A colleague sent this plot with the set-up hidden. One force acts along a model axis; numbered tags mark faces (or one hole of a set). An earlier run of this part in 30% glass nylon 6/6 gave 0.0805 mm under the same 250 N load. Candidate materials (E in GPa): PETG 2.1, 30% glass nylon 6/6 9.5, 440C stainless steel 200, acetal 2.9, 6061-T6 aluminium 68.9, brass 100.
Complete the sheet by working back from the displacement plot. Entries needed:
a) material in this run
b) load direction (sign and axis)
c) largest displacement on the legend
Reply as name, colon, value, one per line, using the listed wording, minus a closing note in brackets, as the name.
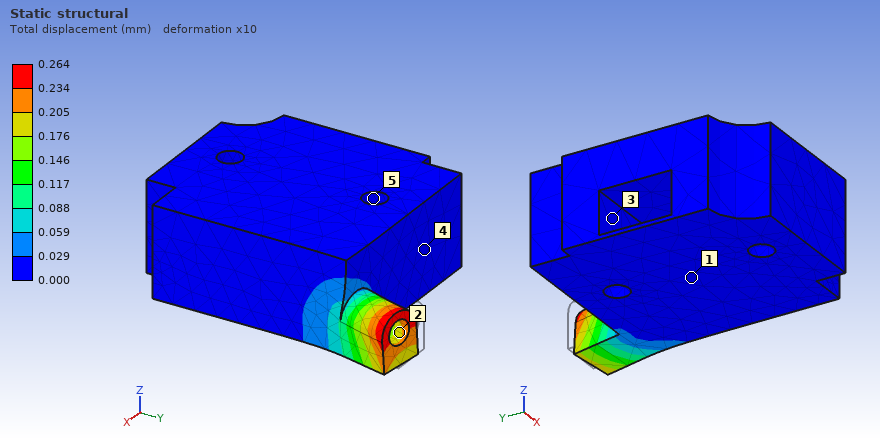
material in this run: acetal
load direction: +X
largest displacement on the legend: 0.264 mm
